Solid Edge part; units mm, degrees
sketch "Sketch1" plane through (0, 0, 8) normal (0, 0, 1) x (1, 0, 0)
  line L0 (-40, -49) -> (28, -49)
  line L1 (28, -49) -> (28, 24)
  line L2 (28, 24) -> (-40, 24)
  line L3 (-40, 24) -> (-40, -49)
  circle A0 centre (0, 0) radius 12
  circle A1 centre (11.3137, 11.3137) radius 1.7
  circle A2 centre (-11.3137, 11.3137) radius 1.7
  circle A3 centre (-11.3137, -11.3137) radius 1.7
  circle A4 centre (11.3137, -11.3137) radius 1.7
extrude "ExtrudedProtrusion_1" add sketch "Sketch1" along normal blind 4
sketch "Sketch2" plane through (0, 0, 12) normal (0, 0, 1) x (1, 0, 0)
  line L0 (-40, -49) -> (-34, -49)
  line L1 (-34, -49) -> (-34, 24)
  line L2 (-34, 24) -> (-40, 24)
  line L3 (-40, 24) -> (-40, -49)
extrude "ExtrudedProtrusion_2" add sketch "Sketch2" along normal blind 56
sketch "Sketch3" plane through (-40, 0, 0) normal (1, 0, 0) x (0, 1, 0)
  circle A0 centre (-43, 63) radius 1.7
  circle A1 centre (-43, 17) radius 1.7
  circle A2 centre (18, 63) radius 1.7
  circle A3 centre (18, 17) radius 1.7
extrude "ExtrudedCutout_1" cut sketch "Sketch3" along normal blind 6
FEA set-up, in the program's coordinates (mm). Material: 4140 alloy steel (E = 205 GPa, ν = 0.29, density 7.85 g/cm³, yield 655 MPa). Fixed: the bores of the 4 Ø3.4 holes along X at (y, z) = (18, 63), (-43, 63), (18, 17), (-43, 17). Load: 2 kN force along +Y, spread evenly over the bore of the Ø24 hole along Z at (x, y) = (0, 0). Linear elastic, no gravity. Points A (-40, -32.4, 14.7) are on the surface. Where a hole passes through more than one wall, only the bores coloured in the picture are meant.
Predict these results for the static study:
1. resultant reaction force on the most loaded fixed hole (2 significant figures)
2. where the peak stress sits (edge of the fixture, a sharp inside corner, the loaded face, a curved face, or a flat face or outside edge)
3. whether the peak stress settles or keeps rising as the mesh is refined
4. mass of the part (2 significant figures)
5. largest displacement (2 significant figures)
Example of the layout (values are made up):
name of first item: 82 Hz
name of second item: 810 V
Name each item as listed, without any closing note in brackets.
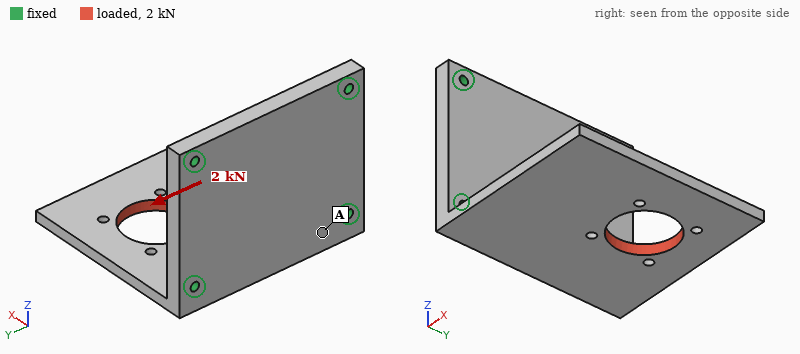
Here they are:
resultant reaction force on the most loaded fixed hole: 1.6 kN
where the peak stress sits: edge of the fixture
whether the peak stress settles or keeps rising as the mesh is refined: keeps rising
mass of the part: 330 g
largest displacement: 23 µm
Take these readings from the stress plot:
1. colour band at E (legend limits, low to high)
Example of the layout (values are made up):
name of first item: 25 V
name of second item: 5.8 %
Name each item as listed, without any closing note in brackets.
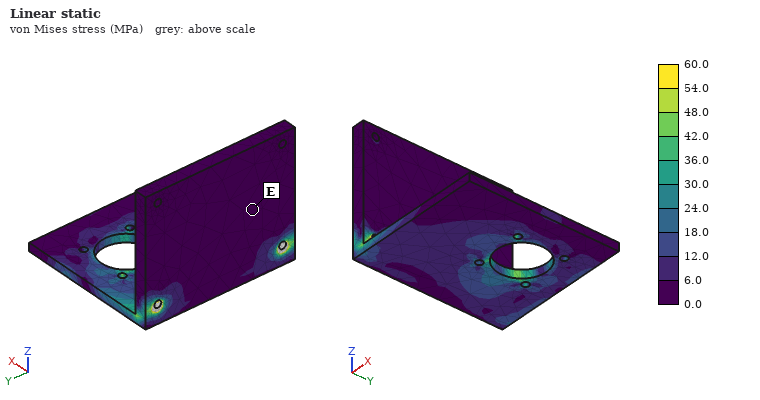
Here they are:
colour band at E: 0.0 to 6.0 MPa
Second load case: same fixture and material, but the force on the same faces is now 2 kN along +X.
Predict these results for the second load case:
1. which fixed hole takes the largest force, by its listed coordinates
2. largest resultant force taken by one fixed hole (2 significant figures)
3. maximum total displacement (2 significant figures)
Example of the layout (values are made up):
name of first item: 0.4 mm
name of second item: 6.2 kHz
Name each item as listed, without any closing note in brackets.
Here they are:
which fixed hole takes the largest force, by its listed coordinates: (18, 17)
largest resultant force taken by one fixed hole: 1.5 kN
maximum total displacement: 30 µm
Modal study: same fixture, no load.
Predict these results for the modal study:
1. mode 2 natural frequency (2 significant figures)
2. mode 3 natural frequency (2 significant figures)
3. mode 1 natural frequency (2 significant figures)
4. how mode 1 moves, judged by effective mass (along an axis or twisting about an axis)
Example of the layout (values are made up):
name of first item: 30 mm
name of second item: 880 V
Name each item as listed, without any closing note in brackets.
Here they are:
mode 2 natural frequency: 1700 Hz
mode 3 natural frequency: 4200 Hz
mode 1 natural frequency: 760 Hz
how mode 1 moves, judged by effective mass: along Z
